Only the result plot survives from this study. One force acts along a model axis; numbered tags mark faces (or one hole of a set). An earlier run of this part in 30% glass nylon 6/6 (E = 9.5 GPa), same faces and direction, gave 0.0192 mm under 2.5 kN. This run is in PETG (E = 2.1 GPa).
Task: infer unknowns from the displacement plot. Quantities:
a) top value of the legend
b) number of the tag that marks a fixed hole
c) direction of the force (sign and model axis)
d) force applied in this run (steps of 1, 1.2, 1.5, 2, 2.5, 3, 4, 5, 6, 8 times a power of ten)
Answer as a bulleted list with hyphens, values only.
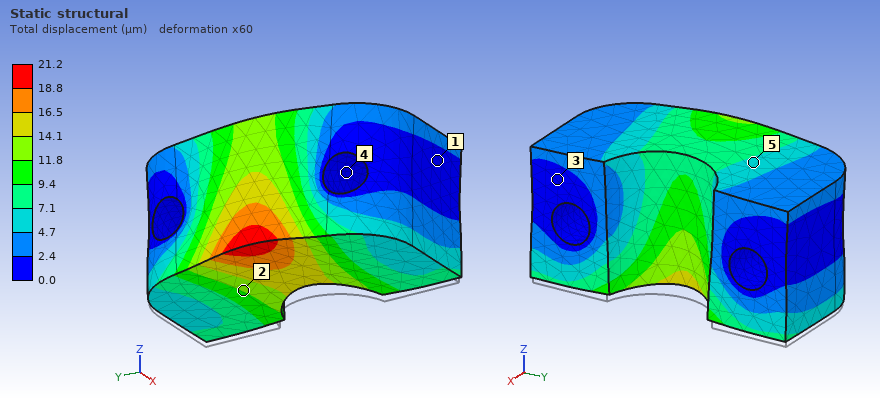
- 21.2 µm
- 4
- +Z
- 600 N
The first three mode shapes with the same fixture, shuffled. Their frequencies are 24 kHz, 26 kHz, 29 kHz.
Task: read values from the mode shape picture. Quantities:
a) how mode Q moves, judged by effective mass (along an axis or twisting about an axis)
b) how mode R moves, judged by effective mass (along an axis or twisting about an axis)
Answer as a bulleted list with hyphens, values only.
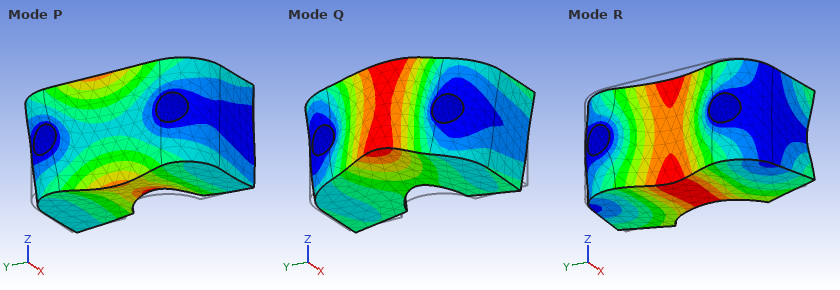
- along Z
- along X
